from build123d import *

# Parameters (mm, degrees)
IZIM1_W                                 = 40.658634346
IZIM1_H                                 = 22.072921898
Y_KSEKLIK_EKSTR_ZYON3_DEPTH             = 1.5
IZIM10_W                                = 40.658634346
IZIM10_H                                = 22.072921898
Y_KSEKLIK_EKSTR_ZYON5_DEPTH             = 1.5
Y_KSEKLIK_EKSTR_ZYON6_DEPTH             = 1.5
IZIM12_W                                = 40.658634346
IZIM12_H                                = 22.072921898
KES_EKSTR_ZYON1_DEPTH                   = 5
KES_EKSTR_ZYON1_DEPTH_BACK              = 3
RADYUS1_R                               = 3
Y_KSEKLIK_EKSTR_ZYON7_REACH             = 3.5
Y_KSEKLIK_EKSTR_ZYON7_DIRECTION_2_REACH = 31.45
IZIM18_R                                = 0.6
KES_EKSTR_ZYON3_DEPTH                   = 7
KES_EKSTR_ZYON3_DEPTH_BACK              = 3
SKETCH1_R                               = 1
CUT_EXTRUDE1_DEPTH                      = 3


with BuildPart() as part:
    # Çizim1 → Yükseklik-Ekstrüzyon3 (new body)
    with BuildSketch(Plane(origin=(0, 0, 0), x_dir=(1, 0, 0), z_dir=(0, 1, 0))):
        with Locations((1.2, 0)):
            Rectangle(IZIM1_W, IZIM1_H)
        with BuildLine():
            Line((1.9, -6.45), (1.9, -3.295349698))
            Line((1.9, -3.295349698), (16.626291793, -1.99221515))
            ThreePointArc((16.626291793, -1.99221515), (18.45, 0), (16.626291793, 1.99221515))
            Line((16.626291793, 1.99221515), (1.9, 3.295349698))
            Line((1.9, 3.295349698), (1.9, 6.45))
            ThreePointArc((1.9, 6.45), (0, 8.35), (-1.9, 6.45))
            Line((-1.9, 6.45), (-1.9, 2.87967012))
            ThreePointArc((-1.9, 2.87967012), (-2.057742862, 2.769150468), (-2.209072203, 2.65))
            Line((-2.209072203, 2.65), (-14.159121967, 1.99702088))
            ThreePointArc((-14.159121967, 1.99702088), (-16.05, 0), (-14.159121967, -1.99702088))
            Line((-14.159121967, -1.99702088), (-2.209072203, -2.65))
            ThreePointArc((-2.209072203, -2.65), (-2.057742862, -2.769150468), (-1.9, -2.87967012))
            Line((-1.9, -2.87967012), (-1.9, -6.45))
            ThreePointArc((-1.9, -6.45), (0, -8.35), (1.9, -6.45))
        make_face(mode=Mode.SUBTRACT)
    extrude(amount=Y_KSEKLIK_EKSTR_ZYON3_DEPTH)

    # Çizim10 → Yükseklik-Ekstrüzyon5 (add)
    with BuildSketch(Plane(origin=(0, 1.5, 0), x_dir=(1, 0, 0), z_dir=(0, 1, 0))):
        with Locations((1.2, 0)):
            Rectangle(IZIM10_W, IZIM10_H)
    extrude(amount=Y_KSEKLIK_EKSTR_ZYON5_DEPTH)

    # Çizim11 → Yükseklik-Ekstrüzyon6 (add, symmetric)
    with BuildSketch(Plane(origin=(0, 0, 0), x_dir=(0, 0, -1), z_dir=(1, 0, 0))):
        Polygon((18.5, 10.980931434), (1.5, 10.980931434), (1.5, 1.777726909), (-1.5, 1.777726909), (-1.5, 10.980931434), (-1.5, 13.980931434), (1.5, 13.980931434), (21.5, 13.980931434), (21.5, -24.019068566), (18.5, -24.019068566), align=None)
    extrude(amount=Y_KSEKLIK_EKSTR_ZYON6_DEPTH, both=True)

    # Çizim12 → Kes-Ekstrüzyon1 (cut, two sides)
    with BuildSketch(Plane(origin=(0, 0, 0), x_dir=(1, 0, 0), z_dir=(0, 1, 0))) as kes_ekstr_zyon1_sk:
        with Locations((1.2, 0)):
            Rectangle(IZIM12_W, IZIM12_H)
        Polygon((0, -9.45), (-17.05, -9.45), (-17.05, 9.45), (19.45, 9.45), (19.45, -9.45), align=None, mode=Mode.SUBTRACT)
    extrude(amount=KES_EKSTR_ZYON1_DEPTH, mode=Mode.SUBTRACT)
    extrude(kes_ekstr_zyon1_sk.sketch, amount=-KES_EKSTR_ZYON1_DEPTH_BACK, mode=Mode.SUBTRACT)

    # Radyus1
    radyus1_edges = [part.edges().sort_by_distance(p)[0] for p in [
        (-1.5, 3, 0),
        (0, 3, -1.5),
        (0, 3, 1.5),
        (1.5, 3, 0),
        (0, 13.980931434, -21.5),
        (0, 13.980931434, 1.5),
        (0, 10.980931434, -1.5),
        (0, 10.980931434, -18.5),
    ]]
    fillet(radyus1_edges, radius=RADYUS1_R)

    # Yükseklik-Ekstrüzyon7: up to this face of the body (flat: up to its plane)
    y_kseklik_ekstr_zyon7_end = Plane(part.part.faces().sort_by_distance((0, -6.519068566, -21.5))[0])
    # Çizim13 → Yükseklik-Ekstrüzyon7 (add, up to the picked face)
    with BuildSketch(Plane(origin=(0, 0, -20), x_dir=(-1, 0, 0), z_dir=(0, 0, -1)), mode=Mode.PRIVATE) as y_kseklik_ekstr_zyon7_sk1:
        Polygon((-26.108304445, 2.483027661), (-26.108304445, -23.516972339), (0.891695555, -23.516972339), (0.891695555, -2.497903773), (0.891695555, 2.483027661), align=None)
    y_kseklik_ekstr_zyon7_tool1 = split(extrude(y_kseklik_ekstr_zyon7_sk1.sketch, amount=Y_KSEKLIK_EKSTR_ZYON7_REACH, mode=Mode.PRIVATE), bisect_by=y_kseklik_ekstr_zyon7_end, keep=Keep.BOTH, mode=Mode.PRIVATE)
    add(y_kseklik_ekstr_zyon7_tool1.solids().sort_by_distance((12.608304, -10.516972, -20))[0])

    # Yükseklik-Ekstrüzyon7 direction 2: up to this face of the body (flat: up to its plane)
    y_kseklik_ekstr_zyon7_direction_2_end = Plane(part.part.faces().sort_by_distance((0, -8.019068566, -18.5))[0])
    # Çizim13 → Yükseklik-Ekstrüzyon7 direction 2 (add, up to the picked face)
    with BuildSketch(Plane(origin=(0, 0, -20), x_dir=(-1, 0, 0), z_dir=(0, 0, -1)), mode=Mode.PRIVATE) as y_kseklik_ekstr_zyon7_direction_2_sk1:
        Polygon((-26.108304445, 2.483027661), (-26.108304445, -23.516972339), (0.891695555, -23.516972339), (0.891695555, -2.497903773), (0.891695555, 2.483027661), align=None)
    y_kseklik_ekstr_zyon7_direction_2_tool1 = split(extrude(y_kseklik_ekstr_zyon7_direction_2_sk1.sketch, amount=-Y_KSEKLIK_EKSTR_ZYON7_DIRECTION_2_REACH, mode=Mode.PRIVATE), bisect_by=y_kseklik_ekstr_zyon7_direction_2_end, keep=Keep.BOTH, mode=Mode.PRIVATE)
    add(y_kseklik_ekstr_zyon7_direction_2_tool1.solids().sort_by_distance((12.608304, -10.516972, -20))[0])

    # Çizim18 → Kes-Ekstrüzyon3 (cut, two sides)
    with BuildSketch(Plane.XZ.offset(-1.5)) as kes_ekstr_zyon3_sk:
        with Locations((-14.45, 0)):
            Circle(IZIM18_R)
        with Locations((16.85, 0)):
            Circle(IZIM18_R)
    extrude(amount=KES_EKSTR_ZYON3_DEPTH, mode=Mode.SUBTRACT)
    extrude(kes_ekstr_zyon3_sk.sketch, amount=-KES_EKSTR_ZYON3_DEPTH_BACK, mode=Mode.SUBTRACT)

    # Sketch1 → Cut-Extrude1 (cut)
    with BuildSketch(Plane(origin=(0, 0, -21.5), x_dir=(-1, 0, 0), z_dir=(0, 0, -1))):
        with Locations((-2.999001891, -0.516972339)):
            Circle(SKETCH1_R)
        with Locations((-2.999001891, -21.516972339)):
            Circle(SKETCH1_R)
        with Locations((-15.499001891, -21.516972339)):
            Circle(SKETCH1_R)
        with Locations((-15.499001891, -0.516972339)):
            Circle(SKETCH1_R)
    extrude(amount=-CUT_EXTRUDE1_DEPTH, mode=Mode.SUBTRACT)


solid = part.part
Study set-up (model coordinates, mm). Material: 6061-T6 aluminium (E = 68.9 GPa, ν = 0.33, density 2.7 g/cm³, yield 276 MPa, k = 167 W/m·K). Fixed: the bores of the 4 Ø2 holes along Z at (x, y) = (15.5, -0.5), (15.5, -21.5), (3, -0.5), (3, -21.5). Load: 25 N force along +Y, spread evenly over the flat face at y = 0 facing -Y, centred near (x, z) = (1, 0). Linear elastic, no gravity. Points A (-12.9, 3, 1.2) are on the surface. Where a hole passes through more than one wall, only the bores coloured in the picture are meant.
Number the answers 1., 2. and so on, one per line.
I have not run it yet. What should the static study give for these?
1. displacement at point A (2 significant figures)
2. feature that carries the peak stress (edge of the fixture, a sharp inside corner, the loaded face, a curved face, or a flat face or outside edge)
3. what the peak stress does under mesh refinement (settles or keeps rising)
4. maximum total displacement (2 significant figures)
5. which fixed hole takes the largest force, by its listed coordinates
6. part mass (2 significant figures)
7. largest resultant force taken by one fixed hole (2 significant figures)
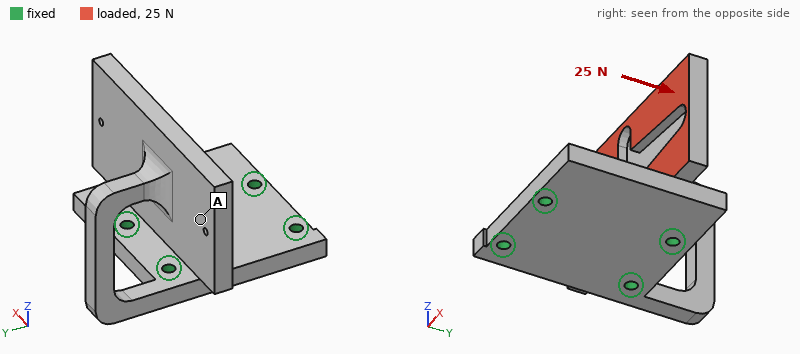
1. 0.35 mm
2. a sharp inside corner
3. keeps rising
4. 0.61 mm
5. (3, -0.5)
6. 12 g
7. 24 N
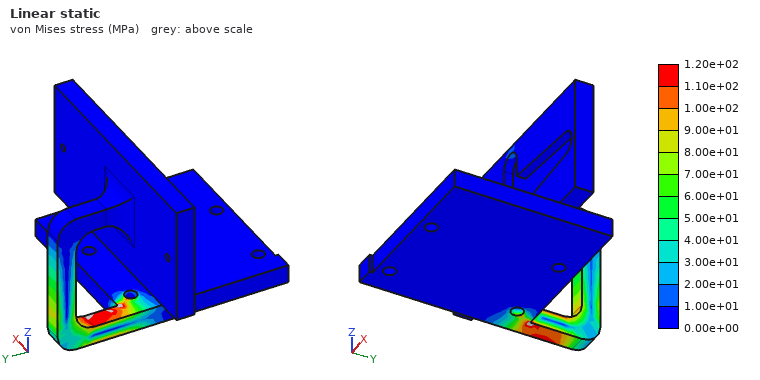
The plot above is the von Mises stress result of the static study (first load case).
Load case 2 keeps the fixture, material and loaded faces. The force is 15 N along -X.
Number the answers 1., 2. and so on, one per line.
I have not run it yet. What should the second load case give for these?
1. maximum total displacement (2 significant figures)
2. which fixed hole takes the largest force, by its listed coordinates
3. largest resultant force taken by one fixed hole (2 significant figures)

1. 0.69 mm
2. (3, -0.5)
3. 15 N
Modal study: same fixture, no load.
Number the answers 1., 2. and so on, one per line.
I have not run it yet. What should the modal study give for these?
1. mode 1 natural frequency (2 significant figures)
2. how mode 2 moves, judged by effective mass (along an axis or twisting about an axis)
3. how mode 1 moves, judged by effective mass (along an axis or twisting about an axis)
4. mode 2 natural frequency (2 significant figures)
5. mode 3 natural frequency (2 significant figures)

1. 380 Hz
2. along Y
3. along X
4. 520 Hz
5. 670 Hz
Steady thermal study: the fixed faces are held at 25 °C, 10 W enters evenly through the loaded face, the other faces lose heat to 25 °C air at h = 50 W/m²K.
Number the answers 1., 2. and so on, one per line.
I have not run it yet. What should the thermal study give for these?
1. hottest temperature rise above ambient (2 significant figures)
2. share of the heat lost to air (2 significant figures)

1. 87 K
2. 68 %
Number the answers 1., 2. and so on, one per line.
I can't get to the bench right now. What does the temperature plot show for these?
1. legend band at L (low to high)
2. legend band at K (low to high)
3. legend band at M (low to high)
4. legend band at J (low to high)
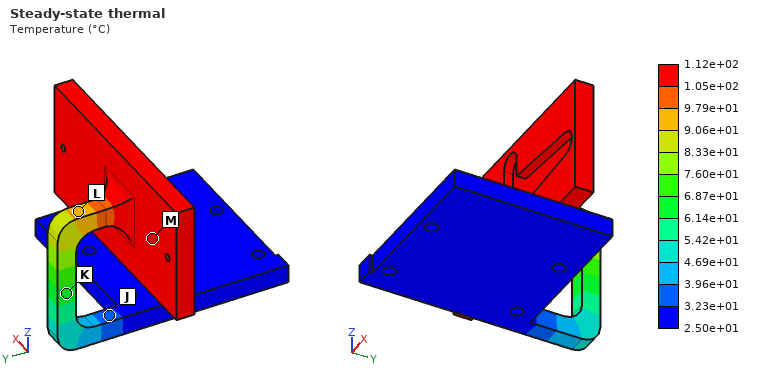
1. 9.06e+01 to 9.79e+01 °C
2. 6.14e+01 to 6.87e+01 °C
3. 1.05e+02 to 1.12e+02 °C
4. 3.23e+01 to 3.96e+01 °C
